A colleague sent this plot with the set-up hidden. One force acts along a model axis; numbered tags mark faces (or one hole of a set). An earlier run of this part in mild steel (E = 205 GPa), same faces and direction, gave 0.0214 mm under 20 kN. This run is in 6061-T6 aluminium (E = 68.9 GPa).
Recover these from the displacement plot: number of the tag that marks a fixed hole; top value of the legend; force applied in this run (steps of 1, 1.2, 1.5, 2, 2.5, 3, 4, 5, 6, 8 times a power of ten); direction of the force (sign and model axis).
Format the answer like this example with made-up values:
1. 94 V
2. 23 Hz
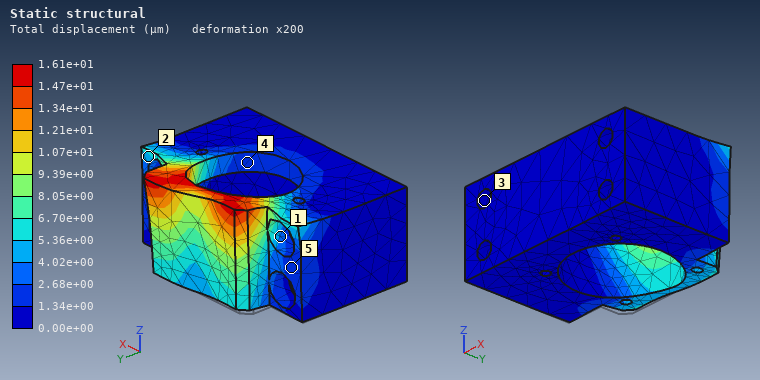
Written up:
1. 3
2. 1.61e+01 µm
3. 5 kN
4. +X
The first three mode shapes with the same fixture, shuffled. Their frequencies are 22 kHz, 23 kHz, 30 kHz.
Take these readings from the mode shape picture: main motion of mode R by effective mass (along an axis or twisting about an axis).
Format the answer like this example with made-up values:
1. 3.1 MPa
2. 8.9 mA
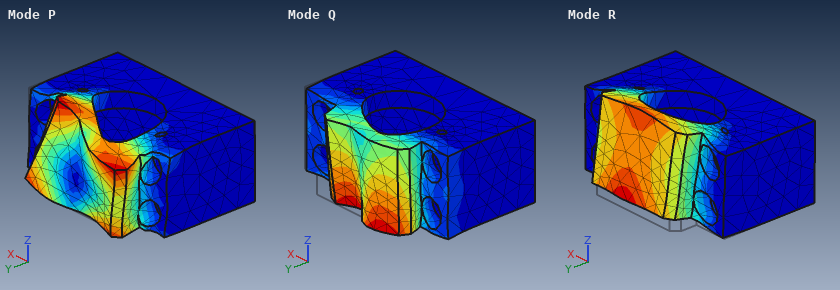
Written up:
1. along Z
